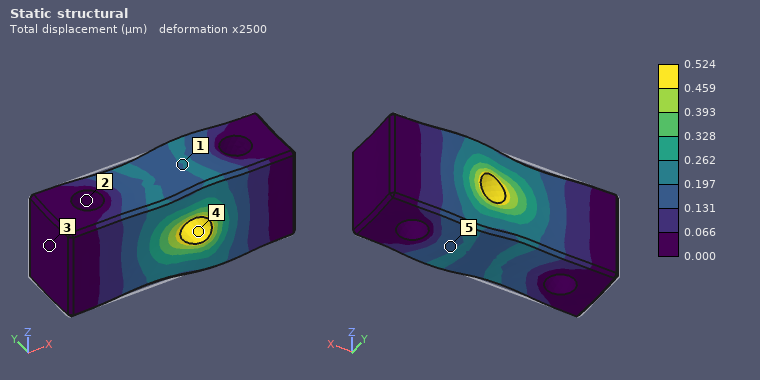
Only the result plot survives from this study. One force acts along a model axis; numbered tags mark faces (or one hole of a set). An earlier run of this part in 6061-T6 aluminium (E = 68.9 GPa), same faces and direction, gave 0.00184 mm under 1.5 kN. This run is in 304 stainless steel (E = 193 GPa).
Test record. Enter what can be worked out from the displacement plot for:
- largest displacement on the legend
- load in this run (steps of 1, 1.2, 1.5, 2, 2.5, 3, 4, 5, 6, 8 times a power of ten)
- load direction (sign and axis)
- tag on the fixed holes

0.524 µm
1.2 kN
+X
2
